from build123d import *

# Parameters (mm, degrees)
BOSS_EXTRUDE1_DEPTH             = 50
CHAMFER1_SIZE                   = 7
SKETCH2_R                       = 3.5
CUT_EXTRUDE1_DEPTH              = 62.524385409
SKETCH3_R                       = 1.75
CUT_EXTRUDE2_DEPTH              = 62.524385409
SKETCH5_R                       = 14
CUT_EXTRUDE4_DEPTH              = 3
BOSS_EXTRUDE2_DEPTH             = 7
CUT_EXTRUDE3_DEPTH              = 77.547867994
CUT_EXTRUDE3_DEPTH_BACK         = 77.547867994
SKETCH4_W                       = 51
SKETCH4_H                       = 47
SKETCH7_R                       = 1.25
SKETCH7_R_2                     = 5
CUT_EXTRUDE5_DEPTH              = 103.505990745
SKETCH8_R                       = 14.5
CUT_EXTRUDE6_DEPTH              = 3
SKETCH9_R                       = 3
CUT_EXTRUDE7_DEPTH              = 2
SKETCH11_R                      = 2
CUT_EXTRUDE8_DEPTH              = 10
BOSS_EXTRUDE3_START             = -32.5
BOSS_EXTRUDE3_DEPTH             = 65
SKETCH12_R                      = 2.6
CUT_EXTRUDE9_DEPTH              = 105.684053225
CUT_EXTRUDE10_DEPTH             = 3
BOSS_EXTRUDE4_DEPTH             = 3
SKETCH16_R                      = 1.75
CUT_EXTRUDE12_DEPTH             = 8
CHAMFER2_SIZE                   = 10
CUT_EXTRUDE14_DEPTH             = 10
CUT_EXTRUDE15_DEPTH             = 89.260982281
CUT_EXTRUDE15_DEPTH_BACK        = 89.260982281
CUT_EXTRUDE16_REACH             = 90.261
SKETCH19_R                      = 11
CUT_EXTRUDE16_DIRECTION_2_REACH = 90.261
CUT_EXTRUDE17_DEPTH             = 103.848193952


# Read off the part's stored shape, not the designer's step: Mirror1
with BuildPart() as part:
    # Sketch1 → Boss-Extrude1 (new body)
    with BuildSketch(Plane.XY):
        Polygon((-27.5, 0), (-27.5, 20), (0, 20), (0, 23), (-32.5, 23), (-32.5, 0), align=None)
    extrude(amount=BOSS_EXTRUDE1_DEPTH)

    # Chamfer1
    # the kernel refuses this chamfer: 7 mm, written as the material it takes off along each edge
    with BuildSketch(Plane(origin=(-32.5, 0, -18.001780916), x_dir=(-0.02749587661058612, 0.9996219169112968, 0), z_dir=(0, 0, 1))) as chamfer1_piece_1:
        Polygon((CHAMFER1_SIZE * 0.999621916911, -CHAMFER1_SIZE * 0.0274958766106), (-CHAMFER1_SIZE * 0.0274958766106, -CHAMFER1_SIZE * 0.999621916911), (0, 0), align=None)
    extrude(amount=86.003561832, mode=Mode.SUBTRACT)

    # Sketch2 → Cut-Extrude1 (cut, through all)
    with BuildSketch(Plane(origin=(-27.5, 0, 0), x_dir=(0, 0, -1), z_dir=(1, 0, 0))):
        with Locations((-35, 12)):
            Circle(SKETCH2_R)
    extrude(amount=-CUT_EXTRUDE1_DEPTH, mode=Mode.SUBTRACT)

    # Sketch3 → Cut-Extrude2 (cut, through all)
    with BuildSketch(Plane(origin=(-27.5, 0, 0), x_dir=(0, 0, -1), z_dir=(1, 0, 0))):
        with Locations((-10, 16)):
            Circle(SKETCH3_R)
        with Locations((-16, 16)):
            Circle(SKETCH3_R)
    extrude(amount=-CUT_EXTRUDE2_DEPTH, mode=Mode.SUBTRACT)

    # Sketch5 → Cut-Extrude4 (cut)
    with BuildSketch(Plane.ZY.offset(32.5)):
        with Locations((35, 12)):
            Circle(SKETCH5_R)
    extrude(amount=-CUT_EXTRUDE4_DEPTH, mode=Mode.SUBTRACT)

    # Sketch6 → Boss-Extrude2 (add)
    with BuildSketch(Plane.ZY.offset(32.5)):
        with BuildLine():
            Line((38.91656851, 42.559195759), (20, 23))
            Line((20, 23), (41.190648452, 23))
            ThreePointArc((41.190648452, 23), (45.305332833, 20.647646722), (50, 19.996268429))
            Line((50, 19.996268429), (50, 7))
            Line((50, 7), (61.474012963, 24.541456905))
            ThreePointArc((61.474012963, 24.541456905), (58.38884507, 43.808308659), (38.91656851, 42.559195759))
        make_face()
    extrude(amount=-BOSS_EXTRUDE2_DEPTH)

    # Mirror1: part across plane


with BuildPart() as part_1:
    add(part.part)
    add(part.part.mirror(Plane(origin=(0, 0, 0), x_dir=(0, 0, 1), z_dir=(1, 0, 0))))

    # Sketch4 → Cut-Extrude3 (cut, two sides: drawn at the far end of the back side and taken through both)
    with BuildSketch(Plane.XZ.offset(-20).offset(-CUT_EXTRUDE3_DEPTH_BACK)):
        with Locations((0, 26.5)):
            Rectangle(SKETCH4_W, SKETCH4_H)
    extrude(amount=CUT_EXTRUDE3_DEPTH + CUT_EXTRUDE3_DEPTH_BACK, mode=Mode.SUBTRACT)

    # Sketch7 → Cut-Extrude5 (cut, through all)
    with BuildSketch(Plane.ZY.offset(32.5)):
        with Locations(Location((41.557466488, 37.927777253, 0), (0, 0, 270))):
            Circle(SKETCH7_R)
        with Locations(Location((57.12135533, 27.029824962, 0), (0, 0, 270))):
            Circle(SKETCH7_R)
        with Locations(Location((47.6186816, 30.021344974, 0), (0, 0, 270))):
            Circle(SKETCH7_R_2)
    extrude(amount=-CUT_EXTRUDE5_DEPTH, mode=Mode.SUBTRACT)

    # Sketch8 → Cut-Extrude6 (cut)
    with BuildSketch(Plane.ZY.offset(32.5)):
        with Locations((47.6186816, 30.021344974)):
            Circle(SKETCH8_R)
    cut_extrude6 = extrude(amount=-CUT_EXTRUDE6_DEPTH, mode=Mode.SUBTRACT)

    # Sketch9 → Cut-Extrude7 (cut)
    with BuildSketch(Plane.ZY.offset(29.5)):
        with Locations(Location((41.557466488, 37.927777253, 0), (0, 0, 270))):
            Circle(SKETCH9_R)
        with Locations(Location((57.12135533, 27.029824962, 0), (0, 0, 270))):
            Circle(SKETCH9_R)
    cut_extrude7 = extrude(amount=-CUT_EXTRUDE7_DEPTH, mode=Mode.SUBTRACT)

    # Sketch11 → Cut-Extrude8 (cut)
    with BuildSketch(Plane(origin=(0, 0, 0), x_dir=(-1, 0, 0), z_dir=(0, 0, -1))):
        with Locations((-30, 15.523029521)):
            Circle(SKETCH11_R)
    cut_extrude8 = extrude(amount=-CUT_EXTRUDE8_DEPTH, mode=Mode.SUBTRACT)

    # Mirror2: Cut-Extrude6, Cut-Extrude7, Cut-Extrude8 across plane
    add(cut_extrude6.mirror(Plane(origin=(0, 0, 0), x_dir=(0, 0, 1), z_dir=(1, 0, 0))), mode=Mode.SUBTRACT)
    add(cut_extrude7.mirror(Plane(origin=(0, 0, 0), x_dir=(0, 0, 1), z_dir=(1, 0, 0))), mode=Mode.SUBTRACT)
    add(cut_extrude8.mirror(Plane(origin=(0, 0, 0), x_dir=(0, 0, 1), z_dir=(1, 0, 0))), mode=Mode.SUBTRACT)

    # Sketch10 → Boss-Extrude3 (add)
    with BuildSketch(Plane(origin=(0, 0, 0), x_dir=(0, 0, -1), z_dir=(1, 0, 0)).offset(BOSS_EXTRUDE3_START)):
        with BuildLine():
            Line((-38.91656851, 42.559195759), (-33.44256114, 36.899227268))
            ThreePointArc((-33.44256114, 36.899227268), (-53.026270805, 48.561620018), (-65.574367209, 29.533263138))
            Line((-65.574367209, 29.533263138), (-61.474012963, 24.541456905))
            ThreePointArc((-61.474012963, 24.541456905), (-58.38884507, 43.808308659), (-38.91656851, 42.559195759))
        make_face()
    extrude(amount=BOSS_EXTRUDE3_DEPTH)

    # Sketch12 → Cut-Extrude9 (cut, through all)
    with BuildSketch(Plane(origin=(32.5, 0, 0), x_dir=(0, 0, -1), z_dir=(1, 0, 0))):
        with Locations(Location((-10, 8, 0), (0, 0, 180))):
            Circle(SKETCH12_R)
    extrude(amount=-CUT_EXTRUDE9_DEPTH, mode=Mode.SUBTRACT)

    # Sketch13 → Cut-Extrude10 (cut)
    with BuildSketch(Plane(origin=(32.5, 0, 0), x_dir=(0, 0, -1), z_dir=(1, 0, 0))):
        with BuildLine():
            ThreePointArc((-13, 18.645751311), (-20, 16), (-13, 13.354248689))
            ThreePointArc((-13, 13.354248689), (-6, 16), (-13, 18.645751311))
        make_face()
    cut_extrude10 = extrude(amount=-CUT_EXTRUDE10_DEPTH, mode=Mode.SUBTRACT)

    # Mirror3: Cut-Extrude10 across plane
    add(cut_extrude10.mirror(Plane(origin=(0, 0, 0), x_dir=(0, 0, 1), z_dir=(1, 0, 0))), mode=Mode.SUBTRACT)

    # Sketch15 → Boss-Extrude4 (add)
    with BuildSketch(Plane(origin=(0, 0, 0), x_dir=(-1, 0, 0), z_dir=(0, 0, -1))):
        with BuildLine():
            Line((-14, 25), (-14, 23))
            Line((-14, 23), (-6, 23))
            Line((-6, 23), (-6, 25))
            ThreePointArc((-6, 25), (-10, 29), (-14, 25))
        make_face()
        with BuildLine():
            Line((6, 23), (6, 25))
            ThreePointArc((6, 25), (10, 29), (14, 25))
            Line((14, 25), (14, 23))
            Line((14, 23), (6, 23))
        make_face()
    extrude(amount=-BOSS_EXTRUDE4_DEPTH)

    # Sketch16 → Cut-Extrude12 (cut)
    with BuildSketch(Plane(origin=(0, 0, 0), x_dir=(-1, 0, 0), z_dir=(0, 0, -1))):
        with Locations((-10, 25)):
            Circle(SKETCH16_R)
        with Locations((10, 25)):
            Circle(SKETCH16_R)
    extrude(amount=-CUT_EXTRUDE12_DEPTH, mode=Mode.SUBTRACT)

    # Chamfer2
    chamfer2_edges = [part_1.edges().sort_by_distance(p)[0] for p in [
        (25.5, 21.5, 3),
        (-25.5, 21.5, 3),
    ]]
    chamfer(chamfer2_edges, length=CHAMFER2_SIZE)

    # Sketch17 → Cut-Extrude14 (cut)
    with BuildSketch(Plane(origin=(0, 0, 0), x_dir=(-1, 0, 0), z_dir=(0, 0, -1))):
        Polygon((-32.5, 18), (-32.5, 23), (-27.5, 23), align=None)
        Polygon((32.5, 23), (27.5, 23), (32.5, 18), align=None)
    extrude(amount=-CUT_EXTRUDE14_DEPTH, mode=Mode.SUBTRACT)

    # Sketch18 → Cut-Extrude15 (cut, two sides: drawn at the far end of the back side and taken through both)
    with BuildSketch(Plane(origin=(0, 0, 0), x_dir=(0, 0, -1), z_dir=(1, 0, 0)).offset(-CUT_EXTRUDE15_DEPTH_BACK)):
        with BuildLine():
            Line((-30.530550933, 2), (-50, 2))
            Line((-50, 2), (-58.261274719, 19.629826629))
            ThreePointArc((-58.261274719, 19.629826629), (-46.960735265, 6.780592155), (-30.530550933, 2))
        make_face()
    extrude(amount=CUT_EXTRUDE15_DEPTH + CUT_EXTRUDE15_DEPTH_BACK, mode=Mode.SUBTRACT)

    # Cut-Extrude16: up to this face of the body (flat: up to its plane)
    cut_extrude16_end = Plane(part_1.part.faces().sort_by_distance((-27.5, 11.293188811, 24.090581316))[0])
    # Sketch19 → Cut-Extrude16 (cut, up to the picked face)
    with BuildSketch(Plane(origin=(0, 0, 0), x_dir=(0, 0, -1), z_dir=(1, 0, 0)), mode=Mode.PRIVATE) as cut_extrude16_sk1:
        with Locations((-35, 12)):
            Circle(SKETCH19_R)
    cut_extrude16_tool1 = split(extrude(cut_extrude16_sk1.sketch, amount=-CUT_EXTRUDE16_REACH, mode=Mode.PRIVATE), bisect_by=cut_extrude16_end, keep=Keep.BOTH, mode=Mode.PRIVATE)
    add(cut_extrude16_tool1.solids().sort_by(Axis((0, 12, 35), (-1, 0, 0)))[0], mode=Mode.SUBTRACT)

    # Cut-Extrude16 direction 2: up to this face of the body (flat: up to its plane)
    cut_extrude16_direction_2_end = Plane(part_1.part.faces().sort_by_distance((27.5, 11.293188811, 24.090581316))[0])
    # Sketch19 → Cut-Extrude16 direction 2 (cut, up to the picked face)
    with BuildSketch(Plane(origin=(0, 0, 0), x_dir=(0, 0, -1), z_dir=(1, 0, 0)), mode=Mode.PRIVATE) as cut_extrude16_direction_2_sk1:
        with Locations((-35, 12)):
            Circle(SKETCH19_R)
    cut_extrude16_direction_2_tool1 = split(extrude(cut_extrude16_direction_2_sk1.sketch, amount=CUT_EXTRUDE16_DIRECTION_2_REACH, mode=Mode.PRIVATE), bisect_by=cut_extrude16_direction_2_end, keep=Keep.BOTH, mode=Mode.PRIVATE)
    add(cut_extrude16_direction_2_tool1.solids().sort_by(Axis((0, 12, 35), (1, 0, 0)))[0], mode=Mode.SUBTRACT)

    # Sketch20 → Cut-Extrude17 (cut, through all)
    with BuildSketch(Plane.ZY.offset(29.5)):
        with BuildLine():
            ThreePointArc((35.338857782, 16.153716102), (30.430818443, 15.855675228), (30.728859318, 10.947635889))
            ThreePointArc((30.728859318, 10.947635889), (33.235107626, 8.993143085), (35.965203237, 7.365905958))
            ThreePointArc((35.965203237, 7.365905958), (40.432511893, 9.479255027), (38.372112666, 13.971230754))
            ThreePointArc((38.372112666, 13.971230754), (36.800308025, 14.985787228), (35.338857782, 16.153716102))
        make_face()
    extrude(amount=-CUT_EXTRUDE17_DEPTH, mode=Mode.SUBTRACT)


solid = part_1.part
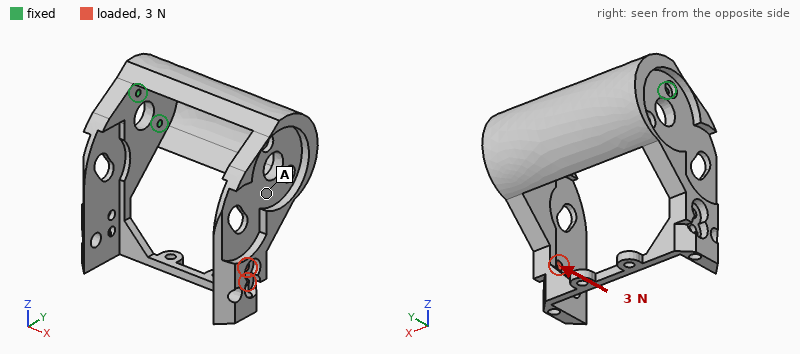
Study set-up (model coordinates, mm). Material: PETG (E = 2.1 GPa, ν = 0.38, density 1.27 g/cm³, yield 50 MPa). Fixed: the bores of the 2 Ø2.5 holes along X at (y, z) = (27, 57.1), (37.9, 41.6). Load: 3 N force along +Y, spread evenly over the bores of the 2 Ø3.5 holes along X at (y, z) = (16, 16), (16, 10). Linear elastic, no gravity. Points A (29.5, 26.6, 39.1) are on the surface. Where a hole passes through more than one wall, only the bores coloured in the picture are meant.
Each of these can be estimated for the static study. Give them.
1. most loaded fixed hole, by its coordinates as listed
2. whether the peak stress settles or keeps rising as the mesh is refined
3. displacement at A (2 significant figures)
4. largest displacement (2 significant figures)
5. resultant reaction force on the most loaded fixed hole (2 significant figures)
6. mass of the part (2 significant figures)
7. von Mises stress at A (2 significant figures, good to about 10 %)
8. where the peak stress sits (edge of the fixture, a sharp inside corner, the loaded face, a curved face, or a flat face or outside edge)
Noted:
(37.9, 41.6)
keeps rising
0.53 mm
1.1 mm
8.1 N
24 g
0.42 MPa
edge of the fixture
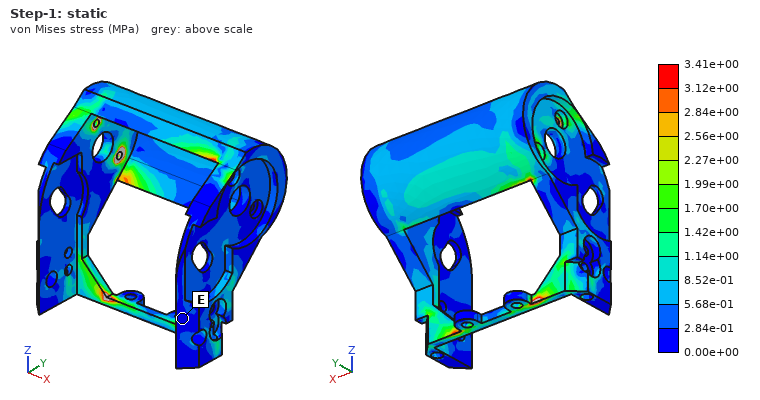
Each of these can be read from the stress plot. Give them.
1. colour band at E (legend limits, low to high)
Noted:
0.00e+00 to 2.84e-01 MPa
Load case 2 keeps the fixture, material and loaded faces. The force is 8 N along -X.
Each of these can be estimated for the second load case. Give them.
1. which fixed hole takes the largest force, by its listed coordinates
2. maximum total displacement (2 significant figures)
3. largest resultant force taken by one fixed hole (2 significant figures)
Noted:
(37.9, 41.6)
1.2 mm
12 N
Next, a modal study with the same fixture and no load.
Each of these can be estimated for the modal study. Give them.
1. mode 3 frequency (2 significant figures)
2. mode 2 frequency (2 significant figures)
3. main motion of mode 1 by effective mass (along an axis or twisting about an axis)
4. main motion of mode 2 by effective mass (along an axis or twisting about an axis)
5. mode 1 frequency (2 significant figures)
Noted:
420 Hz
130 Hz
along Y
along Z
120 Hz
